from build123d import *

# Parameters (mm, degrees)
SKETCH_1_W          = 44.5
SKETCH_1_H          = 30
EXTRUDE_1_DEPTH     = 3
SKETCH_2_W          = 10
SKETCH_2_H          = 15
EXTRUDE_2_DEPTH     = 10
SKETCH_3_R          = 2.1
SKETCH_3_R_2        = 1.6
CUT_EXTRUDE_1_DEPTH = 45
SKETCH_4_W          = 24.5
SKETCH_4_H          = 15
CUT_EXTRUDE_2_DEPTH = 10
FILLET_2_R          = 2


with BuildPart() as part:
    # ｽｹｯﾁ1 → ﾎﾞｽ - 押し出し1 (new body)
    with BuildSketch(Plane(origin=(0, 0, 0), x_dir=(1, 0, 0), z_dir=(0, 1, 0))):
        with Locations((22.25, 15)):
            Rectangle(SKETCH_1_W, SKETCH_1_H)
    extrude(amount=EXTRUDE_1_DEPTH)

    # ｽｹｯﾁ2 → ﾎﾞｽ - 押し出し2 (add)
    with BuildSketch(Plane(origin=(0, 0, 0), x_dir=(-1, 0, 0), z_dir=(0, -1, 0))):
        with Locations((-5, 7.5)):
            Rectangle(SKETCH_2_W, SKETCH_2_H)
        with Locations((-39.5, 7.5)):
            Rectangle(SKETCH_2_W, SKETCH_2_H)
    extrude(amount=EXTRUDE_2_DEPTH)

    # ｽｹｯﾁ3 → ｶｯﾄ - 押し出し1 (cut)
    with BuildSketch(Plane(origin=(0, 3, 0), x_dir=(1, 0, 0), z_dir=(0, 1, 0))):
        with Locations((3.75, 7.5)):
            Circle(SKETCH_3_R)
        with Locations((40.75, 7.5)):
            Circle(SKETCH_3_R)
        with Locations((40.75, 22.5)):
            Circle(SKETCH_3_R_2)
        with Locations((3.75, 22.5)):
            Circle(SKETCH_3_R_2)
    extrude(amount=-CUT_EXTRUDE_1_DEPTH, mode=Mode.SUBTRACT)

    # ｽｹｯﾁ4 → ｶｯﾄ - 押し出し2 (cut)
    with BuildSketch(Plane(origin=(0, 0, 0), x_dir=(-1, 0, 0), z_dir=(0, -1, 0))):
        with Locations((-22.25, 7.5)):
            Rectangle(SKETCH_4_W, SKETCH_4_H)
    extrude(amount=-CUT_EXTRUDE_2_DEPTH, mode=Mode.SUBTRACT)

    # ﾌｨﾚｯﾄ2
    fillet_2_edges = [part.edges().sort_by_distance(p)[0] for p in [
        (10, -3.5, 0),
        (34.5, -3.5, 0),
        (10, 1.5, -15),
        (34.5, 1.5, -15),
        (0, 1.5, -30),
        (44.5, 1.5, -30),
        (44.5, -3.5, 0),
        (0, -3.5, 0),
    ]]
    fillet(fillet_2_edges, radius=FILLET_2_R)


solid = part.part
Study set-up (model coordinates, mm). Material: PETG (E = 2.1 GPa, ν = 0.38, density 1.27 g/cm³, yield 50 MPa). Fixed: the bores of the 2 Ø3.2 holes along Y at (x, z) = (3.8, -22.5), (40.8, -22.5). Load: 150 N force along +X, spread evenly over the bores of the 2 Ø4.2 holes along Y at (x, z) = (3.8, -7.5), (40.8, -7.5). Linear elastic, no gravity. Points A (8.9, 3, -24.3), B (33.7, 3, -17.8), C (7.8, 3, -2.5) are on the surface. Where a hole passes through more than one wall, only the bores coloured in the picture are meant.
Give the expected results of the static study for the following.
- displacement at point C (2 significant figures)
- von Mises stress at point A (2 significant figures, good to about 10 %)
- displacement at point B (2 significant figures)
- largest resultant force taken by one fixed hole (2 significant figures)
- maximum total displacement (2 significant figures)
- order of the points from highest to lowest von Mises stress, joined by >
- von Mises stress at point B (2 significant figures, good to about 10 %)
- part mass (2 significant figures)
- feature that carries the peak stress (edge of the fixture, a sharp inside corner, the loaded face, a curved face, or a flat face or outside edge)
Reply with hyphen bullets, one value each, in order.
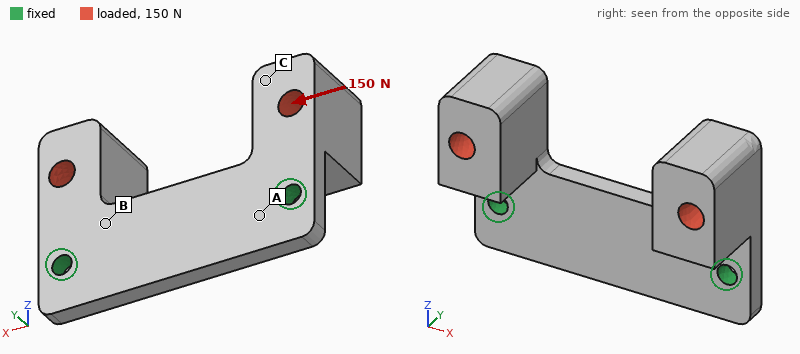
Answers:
- 0.13 mm
- 5.5 MPa
- 0.071 mm
- 91 N
- 0.44 mm
- B > A > C
- 9.1 MPa
- 6.9 g
- a curved face
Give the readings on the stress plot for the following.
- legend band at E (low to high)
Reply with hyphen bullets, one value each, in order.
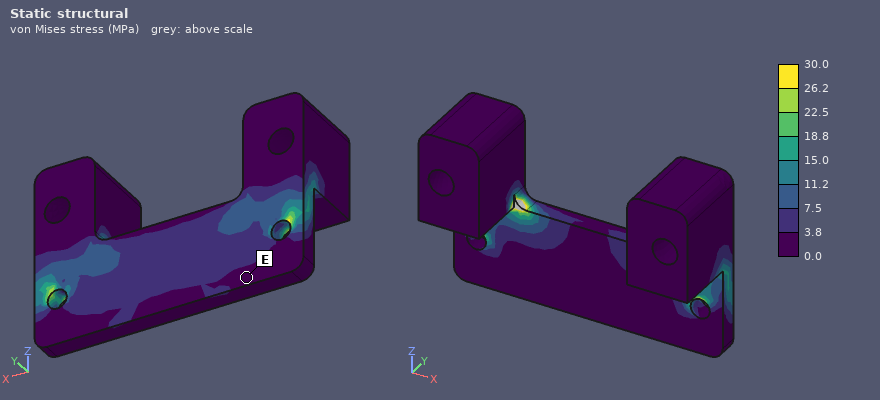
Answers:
- 0.0 to 3.8 MPa
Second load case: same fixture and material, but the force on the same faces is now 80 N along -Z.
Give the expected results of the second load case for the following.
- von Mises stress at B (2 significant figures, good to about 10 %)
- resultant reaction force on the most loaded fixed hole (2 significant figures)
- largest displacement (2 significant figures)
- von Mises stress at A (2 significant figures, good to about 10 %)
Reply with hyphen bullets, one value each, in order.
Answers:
- 6.4 MPa
- 40 N
- 0.63 mm
- 2.3 MPa
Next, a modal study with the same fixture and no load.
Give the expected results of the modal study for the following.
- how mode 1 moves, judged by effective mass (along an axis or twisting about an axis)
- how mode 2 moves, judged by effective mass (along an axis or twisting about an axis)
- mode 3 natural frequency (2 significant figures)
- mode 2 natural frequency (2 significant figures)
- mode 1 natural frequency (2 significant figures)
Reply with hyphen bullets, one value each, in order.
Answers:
- along Y
- twisting about Z
- 1400 Hz
- 700 Hz
- 670 Hz
